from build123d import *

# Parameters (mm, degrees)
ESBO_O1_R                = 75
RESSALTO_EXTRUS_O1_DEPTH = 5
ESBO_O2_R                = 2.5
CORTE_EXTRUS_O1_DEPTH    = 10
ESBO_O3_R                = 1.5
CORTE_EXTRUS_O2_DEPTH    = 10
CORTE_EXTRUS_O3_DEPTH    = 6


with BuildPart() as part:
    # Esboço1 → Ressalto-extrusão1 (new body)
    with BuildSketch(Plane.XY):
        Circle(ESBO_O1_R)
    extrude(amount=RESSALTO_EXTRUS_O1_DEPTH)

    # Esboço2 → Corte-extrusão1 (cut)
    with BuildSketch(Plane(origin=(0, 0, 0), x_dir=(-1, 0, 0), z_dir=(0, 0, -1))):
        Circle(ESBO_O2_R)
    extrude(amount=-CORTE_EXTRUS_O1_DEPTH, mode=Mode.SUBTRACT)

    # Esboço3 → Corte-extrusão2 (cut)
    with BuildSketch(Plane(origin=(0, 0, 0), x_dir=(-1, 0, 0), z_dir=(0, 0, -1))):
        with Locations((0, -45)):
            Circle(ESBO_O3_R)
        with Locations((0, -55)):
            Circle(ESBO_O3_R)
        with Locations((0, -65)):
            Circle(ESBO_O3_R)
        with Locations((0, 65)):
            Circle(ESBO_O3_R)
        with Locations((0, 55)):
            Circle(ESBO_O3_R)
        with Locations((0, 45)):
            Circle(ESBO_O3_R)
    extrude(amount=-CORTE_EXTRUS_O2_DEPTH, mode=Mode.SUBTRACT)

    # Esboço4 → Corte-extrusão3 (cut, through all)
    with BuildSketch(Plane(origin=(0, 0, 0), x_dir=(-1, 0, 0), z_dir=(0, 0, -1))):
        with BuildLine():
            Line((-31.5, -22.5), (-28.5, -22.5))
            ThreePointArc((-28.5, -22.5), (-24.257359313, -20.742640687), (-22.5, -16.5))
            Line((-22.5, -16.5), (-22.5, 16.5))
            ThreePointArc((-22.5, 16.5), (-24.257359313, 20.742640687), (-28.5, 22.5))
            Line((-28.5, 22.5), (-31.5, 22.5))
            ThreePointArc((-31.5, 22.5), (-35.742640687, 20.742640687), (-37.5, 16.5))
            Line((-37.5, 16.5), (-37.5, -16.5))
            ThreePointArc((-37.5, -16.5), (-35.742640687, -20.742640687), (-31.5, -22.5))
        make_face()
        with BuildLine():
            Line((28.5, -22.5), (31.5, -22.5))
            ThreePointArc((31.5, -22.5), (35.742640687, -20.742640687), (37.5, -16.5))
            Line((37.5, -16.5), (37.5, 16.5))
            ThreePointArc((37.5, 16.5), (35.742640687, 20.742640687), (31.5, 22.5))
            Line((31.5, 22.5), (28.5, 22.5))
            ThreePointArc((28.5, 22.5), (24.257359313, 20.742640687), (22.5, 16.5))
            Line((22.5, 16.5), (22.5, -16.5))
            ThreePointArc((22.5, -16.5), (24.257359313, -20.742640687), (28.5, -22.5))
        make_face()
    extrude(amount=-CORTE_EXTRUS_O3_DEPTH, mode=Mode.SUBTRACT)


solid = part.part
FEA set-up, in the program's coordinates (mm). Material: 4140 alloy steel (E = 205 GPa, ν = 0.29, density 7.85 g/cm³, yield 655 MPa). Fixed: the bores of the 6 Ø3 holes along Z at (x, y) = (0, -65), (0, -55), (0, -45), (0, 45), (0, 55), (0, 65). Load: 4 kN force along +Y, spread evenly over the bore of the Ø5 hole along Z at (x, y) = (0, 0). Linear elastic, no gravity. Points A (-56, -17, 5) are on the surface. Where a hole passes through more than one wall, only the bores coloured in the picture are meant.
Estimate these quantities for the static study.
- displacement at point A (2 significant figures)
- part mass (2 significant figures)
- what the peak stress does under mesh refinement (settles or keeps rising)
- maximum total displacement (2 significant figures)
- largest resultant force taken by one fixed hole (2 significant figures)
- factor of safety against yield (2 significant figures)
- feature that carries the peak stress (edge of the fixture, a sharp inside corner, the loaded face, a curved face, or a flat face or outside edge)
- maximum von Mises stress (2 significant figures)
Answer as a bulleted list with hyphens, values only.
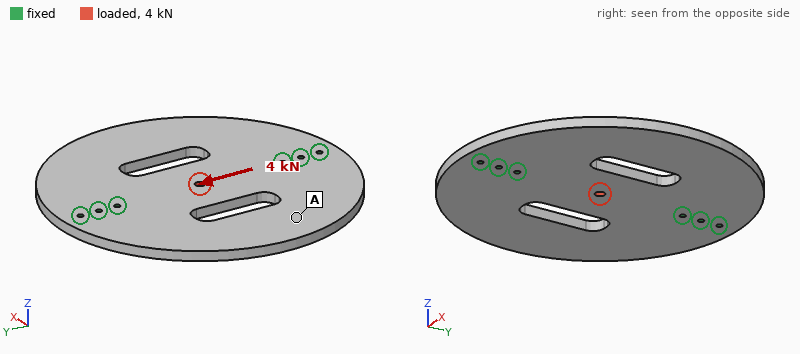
- 1.2 µm
- 640 g
- settles
- 4.1 µm
- 1.2 kN
- 7.5
- the loaded face
- 87 MPa
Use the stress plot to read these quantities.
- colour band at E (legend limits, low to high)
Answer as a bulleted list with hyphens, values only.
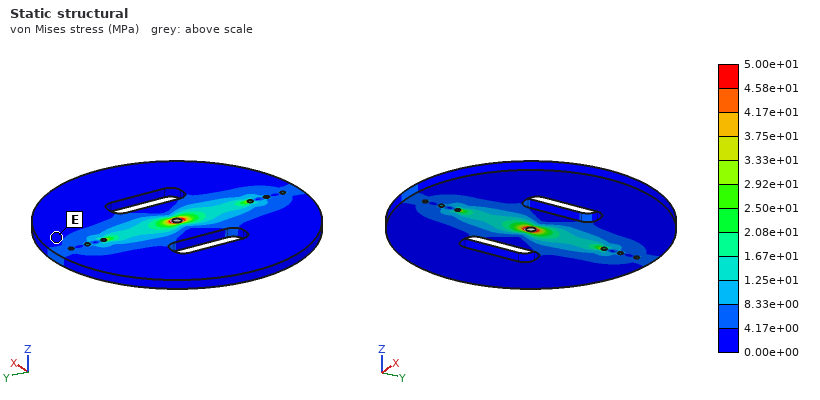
- 0.00e+00 to 4.17e+00 MPa
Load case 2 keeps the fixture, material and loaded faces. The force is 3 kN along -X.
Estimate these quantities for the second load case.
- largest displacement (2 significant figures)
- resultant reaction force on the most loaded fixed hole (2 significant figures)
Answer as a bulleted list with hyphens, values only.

- 5.4 µm
- 1.0 kN
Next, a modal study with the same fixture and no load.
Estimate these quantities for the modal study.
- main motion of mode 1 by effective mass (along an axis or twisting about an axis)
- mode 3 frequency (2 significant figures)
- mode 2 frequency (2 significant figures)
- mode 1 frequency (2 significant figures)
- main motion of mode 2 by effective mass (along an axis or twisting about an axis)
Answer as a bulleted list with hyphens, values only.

- twisting about Y
- 1800 Hz
- 860 Hz
- 690 Hz
- along Z
